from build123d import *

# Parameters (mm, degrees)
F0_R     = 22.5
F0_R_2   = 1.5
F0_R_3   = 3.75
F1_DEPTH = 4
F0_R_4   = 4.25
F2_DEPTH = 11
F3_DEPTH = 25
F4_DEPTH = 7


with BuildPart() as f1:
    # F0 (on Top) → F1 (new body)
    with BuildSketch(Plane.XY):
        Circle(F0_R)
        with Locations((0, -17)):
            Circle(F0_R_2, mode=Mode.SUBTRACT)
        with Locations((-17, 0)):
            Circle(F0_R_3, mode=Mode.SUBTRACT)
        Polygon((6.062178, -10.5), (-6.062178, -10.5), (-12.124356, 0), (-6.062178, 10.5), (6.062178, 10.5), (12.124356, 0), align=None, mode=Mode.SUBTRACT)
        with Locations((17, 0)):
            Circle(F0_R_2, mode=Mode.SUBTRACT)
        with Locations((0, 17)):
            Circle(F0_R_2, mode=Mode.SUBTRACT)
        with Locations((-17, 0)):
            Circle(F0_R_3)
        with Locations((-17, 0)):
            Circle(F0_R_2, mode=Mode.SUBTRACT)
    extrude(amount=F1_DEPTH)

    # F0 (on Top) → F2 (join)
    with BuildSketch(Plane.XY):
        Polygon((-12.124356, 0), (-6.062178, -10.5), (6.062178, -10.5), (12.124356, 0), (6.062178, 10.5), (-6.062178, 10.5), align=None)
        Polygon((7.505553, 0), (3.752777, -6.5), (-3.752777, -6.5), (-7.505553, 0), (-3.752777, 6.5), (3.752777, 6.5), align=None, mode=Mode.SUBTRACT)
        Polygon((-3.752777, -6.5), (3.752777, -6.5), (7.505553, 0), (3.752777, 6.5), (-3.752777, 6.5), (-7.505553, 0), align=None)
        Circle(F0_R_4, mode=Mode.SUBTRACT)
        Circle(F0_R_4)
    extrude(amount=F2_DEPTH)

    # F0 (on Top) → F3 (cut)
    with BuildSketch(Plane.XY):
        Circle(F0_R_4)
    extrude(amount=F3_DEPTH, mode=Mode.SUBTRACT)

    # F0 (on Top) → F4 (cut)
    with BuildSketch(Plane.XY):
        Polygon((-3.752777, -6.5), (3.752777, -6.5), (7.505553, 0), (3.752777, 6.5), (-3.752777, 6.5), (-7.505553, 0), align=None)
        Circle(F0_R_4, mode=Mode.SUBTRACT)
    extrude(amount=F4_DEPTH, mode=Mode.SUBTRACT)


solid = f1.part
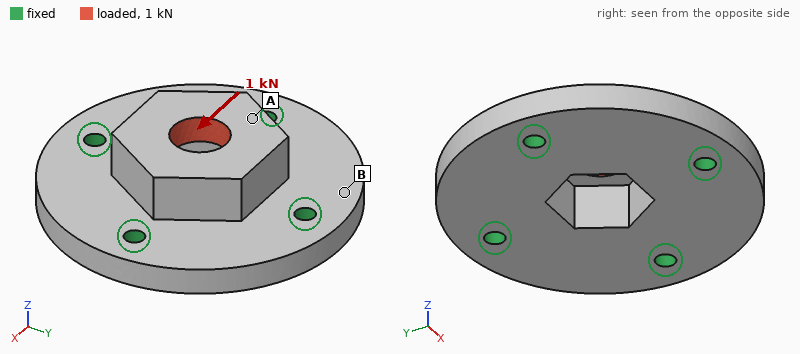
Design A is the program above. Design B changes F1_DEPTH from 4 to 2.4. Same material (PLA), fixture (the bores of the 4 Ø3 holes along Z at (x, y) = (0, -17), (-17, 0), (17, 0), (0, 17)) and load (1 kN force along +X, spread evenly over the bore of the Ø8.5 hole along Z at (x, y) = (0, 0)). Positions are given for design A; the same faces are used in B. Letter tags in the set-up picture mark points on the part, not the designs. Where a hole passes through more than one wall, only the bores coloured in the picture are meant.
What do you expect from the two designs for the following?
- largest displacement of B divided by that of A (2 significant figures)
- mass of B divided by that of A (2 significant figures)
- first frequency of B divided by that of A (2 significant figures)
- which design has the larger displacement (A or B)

2.4
0.75
0.67
B
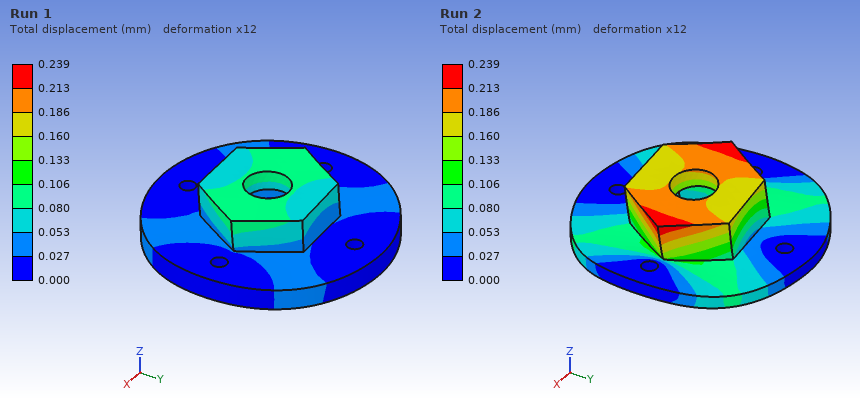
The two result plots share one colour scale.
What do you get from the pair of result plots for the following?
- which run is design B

Run 2
